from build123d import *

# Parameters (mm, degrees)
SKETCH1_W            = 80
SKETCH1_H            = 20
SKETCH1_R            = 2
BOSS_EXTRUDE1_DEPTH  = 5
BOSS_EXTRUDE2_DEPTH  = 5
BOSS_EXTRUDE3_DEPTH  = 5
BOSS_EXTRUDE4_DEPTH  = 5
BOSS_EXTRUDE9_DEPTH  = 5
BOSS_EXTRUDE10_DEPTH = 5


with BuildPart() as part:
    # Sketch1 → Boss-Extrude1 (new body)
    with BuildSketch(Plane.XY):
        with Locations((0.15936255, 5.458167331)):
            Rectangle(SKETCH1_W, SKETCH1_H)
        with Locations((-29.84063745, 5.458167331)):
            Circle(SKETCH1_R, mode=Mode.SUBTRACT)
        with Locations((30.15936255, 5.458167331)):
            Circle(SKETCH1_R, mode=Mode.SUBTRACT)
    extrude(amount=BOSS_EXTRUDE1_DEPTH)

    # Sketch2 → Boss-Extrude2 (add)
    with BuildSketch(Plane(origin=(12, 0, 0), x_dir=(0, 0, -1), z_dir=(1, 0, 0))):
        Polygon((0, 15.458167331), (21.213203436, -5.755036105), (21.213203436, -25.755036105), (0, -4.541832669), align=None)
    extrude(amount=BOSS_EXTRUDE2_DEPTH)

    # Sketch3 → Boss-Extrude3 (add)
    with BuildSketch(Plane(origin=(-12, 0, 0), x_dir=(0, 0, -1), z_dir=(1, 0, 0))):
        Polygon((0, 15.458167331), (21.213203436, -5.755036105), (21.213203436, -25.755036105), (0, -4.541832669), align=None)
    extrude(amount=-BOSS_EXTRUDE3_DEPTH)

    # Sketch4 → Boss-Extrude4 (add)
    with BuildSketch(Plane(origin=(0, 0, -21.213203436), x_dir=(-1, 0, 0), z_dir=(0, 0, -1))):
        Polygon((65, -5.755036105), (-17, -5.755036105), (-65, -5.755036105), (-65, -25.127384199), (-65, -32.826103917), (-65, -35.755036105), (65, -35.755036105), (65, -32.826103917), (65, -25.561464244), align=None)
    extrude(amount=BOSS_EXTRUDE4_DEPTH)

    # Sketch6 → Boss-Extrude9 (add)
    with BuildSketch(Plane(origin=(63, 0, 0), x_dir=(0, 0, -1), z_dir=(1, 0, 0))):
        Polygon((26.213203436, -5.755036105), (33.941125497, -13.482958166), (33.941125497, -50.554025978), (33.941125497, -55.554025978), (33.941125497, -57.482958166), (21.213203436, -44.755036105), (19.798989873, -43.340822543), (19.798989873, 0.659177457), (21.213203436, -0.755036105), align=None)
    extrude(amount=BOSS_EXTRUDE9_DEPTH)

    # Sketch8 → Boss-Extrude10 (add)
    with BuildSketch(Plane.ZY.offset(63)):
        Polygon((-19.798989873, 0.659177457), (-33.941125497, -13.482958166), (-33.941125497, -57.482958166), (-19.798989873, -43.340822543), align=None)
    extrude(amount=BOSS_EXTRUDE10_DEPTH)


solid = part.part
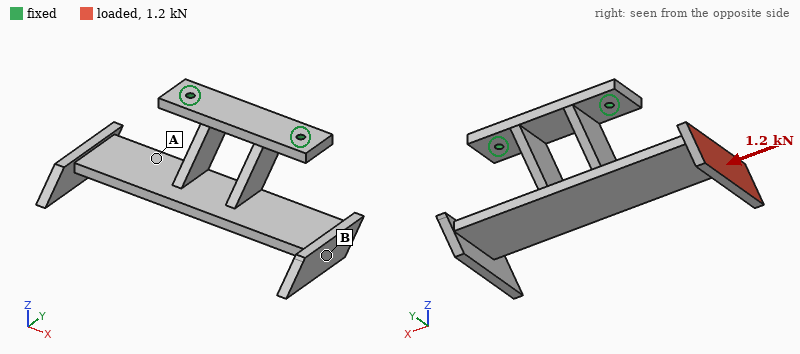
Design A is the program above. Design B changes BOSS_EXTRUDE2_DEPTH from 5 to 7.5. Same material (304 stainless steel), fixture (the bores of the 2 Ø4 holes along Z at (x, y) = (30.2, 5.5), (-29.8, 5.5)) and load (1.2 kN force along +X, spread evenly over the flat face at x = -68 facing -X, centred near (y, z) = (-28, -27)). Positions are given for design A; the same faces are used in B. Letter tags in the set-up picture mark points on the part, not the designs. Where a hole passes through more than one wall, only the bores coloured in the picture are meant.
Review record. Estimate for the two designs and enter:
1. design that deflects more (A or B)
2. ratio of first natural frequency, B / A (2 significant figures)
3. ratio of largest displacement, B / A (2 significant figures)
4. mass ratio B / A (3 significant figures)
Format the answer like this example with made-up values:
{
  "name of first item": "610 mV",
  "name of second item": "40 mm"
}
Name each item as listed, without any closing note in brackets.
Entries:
{
  "design that deflects more": "A",
  "ratio of first natural frequency, B / A": "1.1",
  "ratio of largest displacement, B / A": "0.86",
  "mass ratio B / A": "1.03"
}
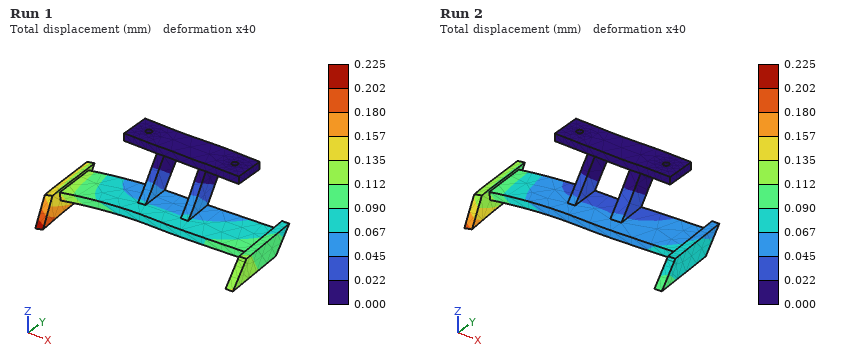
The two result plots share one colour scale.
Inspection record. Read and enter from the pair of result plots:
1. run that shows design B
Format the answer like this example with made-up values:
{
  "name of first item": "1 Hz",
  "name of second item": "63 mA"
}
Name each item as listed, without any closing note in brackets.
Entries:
{
  "run that shows design B": "Run 2"
}
